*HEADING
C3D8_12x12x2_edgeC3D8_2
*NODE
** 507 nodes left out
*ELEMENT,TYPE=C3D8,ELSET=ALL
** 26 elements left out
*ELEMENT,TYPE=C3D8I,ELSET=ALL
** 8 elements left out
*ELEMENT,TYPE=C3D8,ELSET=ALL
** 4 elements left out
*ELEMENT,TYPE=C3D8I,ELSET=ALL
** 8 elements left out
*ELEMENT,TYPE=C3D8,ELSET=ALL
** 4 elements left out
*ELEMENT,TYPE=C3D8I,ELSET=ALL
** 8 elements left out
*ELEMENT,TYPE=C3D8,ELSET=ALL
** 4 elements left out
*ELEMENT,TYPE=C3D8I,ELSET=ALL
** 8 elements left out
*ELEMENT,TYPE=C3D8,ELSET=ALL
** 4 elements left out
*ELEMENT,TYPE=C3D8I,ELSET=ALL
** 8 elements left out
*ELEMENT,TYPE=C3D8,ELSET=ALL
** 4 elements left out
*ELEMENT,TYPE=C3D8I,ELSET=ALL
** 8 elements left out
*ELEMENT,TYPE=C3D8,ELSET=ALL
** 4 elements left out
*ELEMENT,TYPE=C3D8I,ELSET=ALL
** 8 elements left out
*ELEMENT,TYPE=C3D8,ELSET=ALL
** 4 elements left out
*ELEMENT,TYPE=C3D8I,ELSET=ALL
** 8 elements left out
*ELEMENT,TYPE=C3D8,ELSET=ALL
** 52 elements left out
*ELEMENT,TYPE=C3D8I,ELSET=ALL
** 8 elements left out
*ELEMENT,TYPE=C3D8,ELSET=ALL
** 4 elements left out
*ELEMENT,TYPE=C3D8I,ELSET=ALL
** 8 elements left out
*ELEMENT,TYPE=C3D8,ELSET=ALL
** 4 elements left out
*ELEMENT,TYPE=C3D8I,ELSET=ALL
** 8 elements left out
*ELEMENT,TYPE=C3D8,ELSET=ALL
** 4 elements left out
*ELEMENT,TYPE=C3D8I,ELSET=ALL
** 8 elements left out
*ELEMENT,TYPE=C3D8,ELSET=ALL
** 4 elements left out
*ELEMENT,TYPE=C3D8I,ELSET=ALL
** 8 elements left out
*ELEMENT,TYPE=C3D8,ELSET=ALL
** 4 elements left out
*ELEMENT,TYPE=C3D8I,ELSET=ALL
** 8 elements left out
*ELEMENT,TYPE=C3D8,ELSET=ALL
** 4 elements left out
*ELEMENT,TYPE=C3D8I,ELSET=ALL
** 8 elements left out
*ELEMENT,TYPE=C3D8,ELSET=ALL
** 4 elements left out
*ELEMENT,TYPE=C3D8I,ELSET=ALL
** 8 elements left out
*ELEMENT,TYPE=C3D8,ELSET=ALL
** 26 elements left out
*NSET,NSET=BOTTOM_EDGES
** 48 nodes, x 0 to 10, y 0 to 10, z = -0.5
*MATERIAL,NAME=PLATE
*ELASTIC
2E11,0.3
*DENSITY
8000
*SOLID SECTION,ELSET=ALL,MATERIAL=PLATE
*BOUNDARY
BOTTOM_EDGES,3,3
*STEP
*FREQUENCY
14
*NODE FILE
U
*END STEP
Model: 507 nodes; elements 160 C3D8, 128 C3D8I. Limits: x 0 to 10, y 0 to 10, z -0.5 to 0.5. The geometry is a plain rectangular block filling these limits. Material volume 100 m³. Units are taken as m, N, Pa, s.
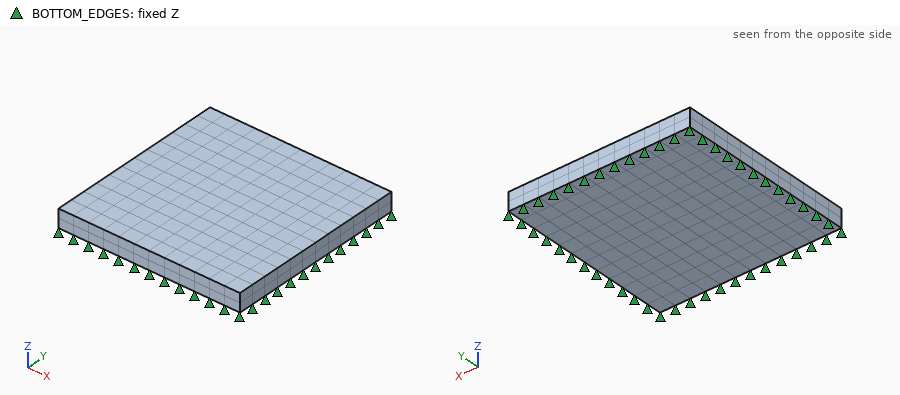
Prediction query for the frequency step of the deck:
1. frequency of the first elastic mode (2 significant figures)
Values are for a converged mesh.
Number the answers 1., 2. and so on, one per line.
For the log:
1. 43 Hz
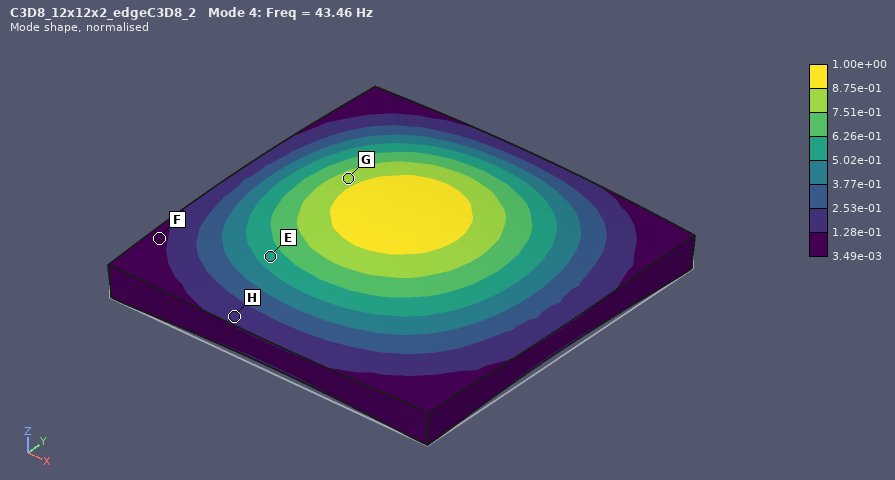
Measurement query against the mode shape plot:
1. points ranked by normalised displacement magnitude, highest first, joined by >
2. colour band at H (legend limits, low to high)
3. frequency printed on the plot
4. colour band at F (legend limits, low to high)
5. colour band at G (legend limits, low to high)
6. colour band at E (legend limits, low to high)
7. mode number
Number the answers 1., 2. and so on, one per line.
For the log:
1. G > E > H > F
2. 1.28e-01 to 2.53e-01
3. 43.46 Hz
4. 3.49e-03 to 1.28e-01
5. 7.51e-01 to 8.75e-01
6. 5.02e-01 to 6.26e-01
7. 4
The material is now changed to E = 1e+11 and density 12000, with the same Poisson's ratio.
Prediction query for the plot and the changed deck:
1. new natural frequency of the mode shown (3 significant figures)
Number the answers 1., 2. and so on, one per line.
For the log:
1. 25.1 Hz
